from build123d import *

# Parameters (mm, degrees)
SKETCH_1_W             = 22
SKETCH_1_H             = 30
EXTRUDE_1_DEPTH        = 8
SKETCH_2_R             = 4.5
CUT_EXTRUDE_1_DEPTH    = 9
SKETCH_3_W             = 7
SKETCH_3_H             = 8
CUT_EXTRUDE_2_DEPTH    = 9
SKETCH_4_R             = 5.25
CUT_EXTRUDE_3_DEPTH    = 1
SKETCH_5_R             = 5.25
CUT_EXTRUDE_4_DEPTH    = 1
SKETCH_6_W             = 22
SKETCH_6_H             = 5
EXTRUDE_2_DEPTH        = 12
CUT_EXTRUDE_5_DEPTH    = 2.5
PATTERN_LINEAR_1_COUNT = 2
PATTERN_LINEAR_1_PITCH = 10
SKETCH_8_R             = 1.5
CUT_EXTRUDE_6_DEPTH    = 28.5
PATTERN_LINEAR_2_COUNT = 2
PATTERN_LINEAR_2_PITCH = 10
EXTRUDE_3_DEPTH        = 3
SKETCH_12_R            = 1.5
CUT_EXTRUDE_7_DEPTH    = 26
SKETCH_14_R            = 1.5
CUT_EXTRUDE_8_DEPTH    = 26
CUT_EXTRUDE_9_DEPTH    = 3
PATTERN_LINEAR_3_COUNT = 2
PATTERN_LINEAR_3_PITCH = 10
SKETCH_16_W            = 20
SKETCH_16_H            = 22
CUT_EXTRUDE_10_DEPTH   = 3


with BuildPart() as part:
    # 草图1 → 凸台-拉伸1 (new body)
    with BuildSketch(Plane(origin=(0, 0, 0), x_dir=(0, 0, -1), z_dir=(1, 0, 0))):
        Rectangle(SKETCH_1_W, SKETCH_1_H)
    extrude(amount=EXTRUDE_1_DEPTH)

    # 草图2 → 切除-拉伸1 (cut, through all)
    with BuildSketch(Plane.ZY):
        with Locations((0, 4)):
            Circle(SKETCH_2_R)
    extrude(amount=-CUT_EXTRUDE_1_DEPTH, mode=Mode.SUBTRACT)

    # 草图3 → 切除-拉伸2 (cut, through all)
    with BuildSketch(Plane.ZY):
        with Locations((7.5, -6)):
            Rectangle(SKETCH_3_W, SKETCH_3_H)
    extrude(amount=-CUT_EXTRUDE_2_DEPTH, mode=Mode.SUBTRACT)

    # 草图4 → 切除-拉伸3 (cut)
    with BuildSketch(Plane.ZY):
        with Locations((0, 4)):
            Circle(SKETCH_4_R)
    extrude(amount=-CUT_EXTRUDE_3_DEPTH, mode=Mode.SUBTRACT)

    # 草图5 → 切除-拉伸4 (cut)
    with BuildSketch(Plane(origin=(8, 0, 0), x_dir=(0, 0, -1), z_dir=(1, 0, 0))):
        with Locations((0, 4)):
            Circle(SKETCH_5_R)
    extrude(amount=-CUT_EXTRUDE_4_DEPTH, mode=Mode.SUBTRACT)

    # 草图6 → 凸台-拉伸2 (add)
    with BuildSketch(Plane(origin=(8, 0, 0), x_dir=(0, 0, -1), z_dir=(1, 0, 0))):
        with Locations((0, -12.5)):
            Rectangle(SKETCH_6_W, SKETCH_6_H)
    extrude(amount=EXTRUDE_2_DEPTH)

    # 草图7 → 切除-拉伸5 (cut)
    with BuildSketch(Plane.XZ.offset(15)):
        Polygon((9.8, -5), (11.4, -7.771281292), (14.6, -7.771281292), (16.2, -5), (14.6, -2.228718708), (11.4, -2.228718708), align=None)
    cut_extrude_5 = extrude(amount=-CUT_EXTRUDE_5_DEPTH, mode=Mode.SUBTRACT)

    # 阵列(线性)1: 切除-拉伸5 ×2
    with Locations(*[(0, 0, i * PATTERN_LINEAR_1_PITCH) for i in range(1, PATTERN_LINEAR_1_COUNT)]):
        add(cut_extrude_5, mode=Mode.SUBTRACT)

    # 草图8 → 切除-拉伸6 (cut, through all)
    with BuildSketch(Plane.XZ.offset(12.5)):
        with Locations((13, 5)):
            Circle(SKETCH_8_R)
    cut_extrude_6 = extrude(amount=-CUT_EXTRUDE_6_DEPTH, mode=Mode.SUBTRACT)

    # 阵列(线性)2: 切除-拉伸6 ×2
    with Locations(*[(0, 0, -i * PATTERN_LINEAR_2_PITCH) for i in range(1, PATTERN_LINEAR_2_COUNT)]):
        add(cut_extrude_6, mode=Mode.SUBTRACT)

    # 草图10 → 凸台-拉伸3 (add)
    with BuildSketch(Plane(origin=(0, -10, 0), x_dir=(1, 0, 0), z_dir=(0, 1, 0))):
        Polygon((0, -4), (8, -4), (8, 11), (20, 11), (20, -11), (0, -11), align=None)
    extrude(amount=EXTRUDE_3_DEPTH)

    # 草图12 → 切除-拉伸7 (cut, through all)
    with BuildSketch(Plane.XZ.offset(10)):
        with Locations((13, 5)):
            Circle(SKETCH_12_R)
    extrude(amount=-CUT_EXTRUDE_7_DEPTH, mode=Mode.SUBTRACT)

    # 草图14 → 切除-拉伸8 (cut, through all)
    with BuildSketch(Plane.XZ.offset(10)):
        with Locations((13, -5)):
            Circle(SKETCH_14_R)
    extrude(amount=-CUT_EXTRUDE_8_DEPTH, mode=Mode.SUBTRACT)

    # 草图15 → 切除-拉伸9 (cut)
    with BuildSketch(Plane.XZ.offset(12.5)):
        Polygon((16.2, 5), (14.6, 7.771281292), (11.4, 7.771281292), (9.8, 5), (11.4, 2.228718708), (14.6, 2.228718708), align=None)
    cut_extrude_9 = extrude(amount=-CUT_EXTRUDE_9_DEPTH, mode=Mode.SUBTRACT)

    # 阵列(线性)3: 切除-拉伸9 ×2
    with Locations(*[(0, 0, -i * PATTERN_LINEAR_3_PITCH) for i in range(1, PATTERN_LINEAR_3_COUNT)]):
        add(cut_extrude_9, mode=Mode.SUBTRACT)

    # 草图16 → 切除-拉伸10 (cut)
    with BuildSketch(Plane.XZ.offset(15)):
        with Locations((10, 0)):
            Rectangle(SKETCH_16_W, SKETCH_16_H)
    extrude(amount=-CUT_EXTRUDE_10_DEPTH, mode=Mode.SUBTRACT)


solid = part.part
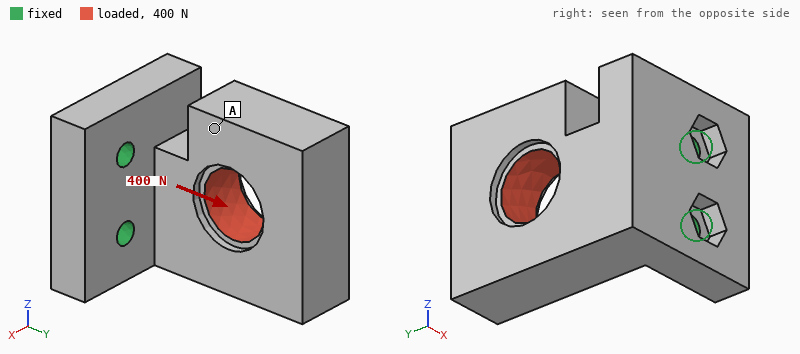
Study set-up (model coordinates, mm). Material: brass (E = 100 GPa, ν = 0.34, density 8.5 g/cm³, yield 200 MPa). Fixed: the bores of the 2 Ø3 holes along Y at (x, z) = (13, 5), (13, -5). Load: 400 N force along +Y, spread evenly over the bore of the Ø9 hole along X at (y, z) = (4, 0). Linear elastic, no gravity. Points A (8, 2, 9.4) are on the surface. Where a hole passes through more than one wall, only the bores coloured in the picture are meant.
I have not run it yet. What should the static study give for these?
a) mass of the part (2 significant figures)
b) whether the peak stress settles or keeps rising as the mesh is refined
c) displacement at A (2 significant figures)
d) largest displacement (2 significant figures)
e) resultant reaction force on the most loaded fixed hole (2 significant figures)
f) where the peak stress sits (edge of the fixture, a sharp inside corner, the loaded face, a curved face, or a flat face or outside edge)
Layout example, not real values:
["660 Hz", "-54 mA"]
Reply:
["43 g", "keeps rising", "20 µm", "47 µm", "200 N", "edge of the fixture"]
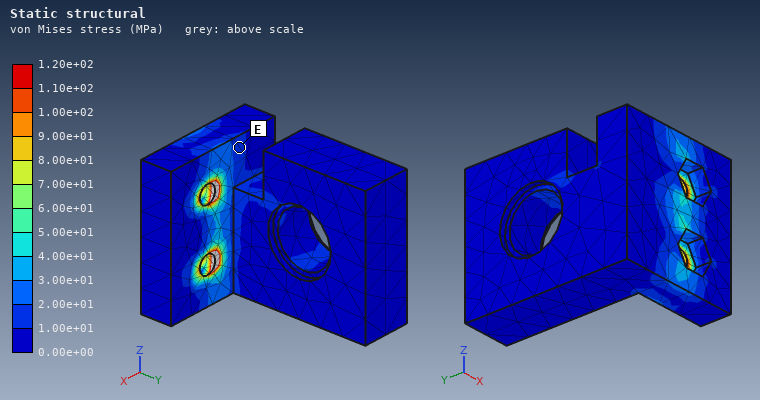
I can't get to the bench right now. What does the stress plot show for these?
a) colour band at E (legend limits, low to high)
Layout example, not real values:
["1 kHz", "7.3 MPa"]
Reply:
["1.00e+01 to 2.00e+01 MPa"]
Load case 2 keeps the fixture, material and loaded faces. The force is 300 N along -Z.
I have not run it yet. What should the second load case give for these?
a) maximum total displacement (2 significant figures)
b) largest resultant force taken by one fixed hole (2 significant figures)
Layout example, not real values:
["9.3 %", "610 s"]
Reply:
["26 µm", "410 N"]
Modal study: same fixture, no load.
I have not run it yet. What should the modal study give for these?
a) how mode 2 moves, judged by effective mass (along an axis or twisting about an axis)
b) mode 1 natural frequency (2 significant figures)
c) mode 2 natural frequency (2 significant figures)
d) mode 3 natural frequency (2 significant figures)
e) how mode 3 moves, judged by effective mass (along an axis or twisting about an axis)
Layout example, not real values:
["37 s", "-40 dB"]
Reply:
["along Z", "2100 Hz", "3700 Hz", "8200 Hz", "along Y"]
